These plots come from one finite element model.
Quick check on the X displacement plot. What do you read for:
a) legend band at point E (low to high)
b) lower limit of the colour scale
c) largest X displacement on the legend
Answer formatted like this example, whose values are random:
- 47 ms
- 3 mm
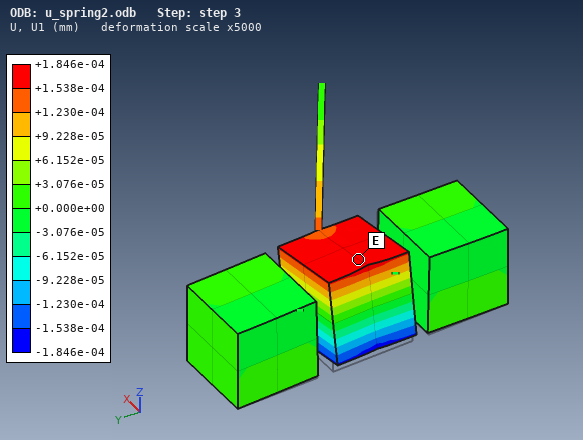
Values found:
- +1.538e-04 to +1.846e-04 mm
- -1.846e-04 mm
- +1.846e-04 mm
